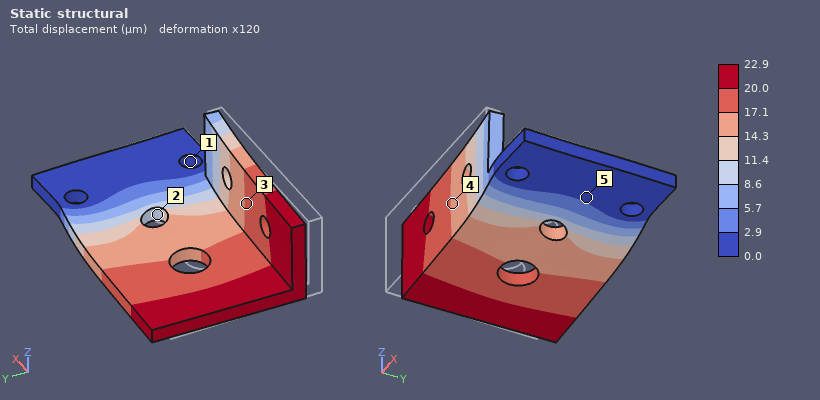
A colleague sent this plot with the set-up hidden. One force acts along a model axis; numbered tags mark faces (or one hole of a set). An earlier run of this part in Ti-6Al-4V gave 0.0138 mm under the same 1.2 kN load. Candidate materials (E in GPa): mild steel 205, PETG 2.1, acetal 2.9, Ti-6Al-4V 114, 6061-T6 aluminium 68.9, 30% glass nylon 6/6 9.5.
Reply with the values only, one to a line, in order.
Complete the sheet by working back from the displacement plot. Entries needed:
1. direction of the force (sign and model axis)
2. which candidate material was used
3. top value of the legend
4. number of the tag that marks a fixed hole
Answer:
+Y
6061-T6 aluminium
22.9 µm
1
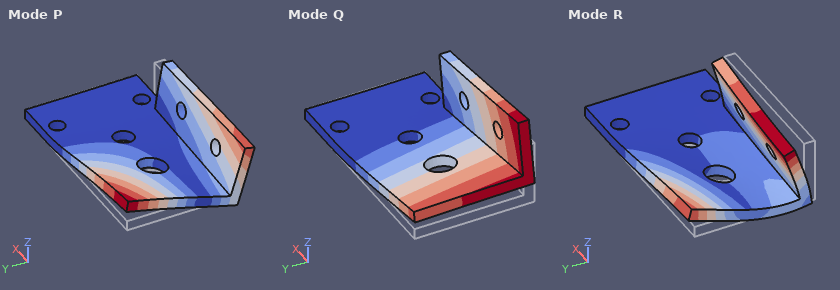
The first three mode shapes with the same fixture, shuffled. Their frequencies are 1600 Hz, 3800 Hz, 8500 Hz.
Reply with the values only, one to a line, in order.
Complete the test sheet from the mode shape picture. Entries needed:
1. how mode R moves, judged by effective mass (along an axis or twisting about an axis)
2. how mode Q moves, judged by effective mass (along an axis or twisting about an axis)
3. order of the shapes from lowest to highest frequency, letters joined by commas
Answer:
along Y
along Z
Q, P, R
